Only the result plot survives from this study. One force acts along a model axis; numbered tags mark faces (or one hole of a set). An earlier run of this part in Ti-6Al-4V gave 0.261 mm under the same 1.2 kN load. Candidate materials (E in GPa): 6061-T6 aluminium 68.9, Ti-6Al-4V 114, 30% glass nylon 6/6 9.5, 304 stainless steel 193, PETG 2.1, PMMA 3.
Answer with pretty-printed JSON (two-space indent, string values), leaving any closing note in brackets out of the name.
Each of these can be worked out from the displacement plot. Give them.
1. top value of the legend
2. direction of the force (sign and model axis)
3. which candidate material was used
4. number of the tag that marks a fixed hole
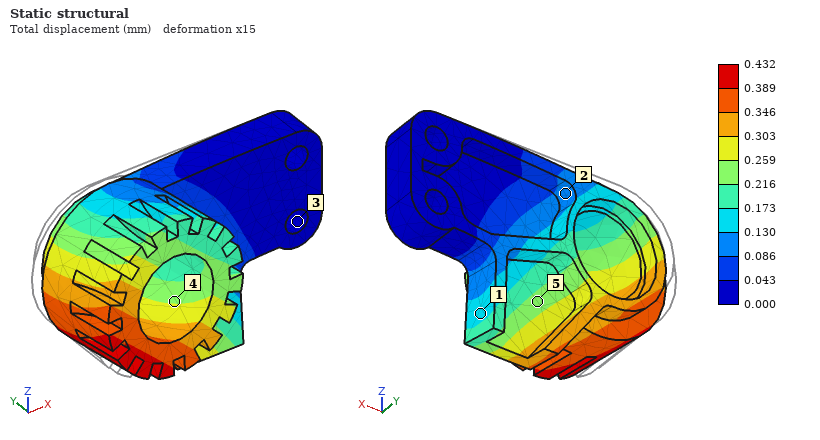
{
  "top value of the legend": "0.432 mm",
  "direction of the force": "-Y",
  "which candidate material was used": "6061-T6 aluminium",
  "number of the tag that marks a fixed hole": "3"
}
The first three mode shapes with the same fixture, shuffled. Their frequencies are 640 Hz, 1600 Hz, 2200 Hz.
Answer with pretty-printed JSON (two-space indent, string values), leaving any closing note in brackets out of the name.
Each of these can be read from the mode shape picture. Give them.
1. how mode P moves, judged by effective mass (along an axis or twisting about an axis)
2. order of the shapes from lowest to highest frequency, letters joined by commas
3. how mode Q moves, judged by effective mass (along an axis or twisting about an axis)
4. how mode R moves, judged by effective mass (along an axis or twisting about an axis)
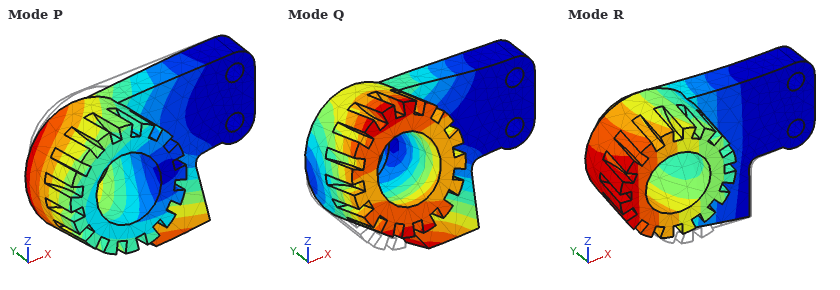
{
  "how mode P moves, judged by effective mass": "along Z",
  "order of the shapes from lowest to highest frequency, letters joined by commas": "R, Q, P",
  "how mode Q moves, judged by effective mass": "along Z",
  "how mode R moves, judged by effective mass": "along Y"
}
